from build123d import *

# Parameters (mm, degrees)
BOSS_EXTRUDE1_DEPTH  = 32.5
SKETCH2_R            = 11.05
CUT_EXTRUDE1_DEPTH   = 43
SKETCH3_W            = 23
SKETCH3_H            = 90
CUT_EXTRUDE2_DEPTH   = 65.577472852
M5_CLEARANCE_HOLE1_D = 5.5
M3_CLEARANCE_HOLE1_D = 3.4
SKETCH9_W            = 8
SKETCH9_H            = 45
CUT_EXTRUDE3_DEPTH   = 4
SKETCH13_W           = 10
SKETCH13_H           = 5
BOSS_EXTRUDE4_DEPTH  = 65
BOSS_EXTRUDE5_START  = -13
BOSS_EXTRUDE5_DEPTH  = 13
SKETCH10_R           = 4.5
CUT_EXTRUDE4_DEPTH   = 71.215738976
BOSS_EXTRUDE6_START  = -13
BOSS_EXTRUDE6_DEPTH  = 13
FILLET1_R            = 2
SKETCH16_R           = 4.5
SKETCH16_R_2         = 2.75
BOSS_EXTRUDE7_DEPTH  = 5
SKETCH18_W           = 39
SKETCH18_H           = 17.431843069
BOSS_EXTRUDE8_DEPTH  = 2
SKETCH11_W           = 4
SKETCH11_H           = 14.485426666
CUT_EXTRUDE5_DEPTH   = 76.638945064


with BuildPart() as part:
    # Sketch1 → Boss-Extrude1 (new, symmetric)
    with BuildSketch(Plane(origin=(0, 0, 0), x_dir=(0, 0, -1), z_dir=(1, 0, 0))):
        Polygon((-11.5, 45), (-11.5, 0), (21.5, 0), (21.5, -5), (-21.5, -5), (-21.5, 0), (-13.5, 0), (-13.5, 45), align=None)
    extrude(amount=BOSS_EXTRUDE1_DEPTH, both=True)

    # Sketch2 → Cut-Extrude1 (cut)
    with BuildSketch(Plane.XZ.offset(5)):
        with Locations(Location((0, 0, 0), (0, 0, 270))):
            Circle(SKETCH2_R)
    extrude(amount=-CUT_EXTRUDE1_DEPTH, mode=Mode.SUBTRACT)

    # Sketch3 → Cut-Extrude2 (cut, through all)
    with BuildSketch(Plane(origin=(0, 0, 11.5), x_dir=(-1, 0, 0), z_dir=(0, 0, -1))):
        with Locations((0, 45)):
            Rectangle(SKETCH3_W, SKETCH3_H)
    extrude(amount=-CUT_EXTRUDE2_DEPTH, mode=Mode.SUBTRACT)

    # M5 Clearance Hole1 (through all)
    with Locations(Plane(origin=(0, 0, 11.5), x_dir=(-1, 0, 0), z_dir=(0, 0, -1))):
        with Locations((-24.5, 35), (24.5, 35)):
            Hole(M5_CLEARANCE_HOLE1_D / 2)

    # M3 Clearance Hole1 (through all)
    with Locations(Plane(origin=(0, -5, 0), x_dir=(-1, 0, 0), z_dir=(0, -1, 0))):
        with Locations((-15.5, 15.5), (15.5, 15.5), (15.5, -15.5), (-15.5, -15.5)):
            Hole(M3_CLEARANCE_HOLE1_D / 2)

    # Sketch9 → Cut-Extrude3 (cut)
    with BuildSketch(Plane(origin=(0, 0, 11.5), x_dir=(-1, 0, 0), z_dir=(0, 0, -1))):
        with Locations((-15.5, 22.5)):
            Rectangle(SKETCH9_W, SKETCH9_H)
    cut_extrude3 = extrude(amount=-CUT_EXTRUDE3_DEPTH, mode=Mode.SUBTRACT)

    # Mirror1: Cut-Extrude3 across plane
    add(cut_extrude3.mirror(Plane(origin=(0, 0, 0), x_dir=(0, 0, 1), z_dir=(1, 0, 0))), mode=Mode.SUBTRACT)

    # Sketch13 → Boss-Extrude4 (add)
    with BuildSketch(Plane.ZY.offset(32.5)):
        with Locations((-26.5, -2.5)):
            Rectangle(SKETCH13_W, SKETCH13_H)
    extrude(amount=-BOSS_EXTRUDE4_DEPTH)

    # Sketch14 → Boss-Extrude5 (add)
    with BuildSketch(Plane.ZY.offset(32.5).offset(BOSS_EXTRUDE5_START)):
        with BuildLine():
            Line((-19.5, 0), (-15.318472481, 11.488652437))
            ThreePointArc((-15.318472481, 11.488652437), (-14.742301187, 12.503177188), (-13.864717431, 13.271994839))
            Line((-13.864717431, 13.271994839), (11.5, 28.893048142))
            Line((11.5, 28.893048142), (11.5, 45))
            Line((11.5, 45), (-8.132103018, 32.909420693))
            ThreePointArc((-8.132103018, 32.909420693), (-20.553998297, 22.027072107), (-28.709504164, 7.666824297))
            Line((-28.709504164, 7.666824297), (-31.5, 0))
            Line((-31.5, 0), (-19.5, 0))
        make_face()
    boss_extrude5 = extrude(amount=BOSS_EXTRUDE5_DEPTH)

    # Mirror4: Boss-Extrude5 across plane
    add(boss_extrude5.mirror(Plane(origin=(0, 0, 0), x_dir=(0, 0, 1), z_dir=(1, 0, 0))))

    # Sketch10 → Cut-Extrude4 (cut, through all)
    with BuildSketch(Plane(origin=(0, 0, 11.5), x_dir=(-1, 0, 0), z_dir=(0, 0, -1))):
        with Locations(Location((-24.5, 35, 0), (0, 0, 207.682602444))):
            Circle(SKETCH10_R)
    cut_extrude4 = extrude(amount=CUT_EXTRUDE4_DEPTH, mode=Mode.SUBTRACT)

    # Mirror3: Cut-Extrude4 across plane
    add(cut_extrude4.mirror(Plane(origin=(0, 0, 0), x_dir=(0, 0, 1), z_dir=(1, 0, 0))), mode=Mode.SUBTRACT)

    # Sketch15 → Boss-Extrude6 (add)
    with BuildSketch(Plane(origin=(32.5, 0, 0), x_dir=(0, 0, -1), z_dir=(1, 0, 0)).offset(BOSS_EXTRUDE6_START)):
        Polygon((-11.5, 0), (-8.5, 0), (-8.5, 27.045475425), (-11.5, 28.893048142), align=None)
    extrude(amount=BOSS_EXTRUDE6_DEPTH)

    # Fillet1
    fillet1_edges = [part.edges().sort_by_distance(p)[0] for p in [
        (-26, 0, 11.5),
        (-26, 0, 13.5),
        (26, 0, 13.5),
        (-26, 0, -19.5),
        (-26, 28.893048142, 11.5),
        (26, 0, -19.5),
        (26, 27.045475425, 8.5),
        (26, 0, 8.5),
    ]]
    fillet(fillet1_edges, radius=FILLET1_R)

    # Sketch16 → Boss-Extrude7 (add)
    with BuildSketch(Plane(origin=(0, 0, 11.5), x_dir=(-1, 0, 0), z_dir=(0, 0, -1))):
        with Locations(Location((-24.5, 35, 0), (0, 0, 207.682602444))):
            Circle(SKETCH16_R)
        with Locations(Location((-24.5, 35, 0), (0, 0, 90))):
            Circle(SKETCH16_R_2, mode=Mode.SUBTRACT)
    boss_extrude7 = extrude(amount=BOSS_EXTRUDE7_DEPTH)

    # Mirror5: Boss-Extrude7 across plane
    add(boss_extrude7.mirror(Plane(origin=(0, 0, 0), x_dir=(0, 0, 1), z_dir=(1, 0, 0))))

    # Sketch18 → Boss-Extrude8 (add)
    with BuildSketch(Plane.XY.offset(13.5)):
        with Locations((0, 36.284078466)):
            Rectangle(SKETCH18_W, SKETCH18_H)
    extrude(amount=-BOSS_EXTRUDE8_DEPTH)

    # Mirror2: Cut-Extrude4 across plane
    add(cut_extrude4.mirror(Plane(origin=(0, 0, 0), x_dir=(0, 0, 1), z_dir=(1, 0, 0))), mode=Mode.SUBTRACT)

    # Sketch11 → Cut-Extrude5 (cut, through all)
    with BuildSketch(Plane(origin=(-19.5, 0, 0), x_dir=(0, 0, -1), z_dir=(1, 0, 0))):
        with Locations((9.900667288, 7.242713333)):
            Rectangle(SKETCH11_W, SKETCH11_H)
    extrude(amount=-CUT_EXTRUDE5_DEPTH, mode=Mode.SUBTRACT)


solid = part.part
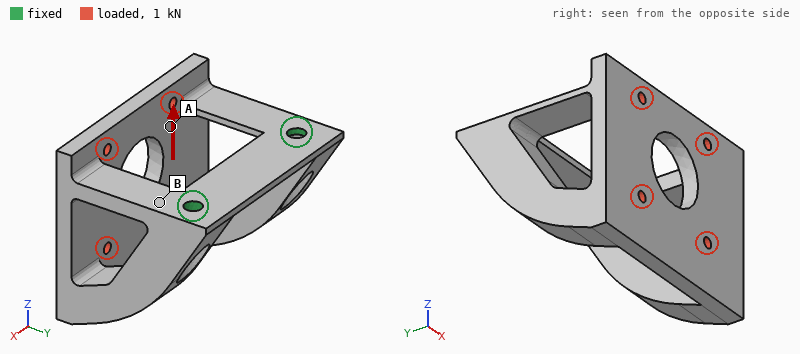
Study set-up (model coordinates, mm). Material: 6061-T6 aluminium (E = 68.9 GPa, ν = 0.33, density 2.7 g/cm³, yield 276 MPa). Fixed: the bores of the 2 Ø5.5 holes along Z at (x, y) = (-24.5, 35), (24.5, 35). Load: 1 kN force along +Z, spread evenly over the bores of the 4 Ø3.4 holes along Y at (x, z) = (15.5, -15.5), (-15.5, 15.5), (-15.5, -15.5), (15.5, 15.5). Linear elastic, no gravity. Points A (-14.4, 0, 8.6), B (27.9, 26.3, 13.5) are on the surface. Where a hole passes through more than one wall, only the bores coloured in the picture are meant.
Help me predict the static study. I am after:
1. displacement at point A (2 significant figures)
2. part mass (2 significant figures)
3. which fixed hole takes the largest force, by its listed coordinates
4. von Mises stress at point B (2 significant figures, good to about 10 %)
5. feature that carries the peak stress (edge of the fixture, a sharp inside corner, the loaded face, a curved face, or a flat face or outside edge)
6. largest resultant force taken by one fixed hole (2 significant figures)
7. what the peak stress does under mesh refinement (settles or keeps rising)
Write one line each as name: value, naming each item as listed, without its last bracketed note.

displacement at point A: 0.20 mm
part mass: 96 g
which fixed hole takes the largest force, by its listed coordinates: (24.5, 35)
von Mises stress at point B: 58 MPa
feature that carries the peak stress: edge of the fixture
largest resultant force taken by one fixed hole: 650 N
what the peak stress does under mesh refinement: keeps rising
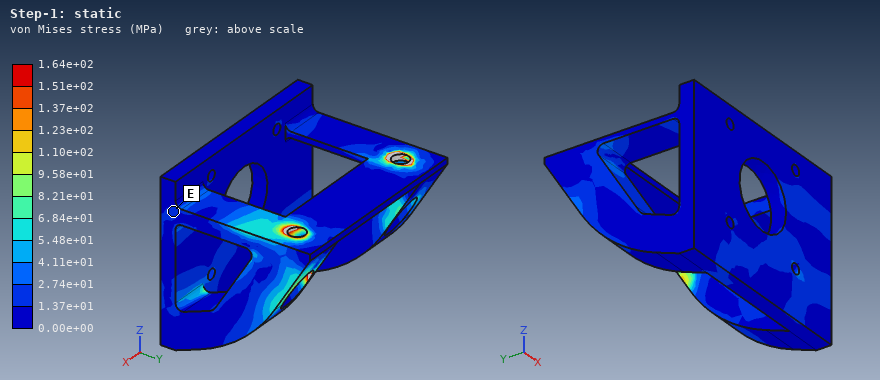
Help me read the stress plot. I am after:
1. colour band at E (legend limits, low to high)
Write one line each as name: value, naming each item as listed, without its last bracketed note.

colour band at E: 1.37e+01 to 2.74e+01 MPa
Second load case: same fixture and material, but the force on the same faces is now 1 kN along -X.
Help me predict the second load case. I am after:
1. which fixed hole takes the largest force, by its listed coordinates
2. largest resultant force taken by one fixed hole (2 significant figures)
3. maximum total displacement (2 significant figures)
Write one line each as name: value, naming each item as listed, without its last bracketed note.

which fixed hole takes the largest force, by its listed coordinates: (24.5, 35)
largest resultant force taken by one fixed hole: 770 N
maximum total displacement: 85 µm
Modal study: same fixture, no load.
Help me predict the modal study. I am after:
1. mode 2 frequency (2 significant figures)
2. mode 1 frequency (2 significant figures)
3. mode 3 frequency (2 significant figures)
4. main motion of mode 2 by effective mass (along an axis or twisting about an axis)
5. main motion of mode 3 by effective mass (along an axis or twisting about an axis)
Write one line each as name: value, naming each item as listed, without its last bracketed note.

mode 2 frequency: 2000 Hz
mode 1 frequency: 1300 Hz
mode 3 frequency: 2800 Hz
main motion of mode 2 by effective mass: along X
main motion of mode 3 by effective mass: along X
